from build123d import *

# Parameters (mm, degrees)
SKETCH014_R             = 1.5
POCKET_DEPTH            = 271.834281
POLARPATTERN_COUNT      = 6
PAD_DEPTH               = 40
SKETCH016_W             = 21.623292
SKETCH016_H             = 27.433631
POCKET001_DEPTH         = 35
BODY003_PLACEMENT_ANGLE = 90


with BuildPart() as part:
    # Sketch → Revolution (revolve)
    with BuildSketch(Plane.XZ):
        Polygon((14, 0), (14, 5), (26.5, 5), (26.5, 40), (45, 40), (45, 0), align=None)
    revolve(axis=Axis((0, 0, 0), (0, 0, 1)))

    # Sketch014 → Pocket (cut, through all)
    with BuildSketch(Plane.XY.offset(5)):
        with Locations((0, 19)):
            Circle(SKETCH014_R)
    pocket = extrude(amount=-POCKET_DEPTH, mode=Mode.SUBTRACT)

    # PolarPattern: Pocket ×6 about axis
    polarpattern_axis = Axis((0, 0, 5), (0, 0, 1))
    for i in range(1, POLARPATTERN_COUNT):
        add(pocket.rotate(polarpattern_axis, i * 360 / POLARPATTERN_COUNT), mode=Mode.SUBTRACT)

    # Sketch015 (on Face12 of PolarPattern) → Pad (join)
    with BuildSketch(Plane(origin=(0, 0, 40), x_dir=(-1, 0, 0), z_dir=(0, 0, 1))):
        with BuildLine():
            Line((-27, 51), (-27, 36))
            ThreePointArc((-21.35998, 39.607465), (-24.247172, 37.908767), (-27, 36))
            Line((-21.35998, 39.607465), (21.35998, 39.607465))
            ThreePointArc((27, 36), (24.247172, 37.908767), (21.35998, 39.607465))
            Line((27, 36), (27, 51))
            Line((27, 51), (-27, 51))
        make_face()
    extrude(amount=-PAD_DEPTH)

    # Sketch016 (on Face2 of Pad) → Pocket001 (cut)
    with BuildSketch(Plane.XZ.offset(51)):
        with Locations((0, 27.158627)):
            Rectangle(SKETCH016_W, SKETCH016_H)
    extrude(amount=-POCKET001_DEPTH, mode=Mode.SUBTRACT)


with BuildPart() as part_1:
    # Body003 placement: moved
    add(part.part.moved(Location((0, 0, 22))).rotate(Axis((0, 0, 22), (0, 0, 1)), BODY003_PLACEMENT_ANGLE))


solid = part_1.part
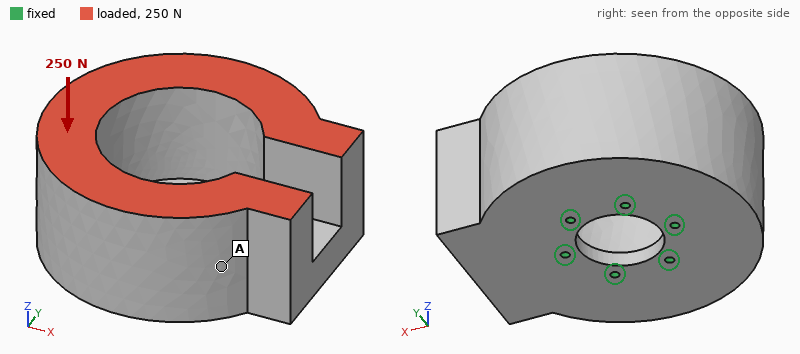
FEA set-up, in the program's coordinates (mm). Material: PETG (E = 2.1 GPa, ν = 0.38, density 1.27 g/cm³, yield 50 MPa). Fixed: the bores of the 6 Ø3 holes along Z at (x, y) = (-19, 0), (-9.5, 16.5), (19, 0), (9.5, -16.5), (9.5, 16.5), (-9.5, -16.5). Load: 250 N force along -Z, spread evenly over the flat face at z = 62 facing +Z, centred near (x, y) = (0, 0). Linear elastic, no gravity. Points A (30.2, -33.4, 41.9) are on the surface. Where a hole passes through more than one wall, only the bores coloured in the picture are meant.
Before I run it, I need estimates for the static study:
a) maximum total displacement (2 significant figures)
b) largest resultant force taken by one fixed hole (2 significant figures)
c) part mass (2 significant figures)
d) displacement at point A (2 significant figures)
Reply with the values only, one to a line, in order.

34 µm
49 N
230 g
26 µm
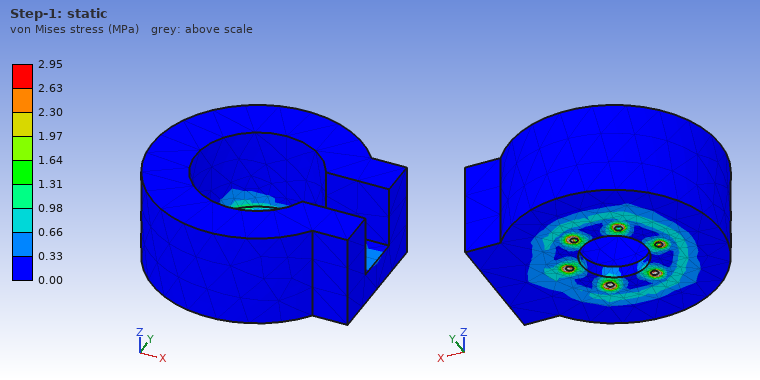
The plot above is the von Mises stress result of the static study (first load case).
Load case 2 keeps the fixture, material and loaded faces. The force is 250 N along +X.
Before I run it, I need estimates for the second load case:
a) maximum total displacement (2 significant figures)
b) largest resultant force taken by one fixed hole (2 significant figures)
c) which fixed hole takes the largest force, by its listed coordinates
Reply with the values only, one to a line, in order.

0.22 mm
140 N
(-19, 0)
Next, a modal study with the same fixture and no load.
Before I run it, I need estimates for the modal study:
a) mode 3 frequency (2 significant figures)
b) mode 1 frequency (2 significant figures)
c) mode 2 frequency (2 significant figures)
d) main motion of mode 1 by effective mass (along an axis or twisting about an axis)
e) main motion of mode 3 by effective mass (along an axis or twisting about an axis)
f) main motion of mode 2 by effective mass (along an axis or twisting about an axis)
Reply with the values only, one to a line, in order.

1200 Hz
560 Hz
600 Hz
along X
along Z
along Y
